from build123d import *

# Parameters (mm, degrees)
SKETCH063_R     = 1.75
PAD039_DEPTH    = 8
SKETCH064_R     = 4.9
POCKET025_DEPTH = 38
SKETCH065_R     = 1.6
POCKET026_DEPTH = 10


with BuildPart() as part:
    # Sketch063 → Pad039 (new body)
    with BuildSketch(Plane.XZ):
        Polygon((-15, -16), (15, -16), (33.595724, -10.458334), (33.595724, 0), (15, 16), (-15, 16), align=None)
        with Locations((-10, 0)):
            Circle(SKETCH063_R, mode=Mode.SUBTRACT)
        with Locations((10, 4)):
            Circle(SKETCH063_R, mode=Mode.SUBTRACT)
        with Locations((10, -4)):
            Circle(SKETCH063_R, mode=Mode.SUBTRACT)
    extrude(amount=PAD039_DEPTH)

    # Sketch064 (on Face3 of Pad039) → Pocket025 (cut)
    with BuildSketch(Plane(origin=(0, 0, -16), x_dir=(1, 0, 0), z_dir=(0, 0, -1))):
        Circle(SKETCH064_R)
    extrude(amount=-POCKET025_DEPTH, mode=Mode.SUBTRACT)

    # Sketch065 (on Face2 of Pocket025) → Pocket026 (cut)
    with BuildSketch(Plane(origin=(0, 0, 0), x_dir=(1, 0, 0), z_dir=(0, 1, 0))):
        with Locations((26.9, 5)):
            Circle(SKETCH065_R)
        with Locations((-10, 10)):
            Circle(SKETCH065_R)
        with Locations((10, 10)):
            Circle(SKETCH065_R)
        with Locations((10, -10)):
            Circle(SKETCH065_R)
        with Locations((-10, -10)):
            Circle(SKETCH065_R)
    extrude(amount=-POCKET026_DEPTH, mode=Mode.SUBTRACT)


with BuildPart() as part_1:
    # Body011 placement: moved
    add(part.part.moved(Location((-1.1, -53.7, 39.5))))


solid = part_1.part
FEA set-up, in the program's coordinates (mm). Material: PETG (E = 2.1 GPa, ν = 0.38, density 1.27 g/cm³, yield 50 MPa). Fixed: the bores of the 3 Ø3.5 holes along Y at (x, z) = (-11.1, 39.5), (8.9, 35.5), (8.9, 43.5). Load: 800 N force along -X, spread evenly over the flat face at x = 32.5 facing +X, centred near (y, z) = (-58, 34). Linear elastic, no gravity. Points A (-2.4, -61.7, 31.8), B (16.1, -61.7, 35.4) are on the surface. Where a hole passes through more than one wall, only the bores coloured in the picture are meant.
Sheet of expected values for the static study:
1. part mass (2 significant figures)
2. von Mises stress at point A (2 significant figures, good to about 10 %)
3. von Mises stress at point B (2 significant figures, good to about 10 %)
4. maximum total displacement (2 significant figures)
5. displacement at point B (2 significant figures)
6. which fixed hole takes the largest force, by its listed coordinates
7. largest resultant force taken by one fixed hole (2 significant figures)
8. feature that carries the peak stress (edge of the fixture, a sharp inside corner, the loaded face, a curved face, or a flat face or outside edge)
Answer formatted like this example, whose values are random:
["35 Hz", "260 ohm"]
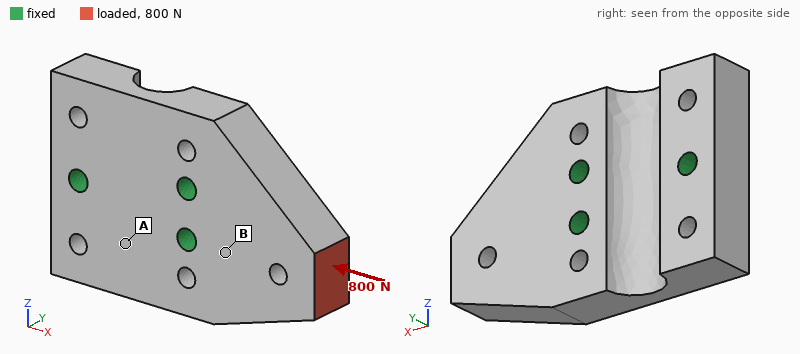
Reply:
["12 g", "2.8 MPa", "7.4 MPa", "0.12 mm", "0.028 mm", "(8.9, 35.5)", "620 N", "a curved face"]
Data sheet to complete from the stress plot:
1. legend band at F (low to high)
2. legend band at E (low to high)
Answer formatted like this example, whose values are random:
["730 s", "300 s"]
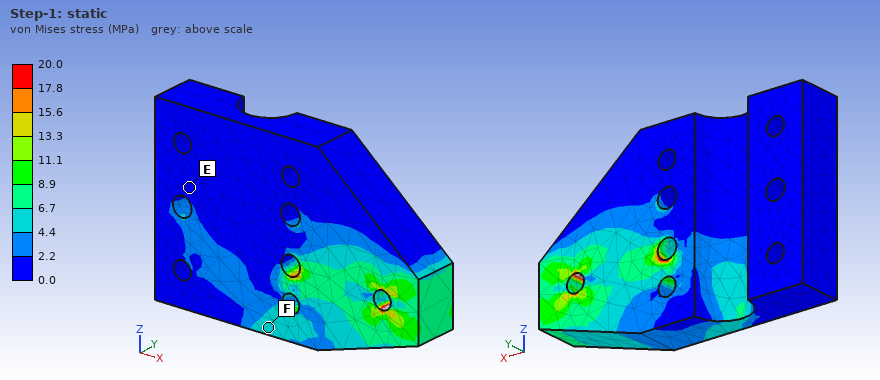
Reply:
["4.4 to 6.7 MPa", "0.0 to 2.2 MPa"]
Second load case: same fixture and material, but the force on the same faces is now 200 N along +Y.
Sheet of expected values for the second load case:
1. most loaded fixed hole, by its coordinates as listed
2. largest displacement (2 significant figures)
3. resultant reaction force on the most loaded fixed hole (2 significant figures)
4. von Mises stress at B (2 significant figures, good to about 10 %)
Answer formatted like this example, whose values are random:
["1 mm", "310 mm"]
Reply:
["(8.9, 35.5)", "0.54 mm", "170 N", "13 MPa"]
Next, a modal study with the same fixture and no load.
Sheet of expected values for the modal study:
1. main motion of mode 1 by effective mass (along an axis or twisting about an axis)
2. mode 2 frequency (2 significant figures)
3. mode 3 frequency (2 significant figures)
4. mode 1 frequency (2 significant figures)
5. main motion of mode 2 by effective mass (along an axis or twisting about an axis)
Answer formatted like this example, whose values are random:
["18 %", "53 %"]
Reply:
["along Y", "5400 Hz", "5900 Hz", "3400 Hz", "along Z"]
